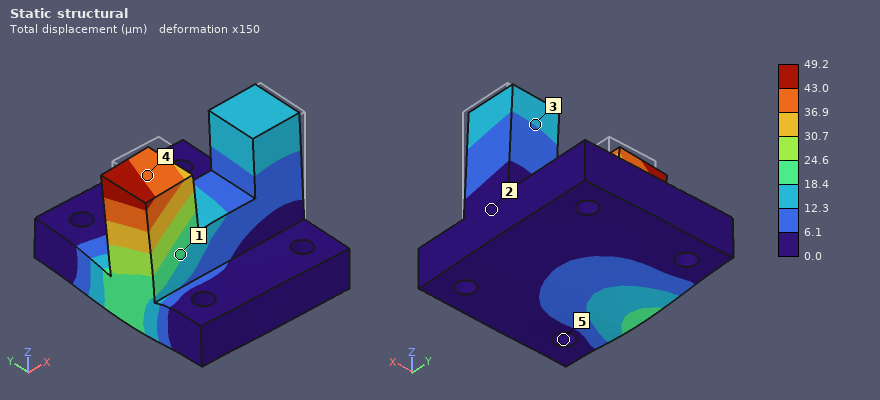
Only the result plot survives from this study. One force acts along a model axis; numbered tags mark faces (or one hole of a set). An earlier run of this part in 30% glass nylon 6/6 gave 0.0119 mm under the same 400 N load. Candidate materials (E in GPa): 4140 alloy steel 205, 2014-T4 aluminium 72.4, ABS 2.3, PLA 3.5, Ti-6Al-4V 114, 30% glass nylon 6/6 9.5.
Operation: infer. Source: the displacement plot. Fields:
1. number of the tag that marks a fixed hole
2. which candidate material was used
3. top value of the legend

5
ABS
49.2 µm
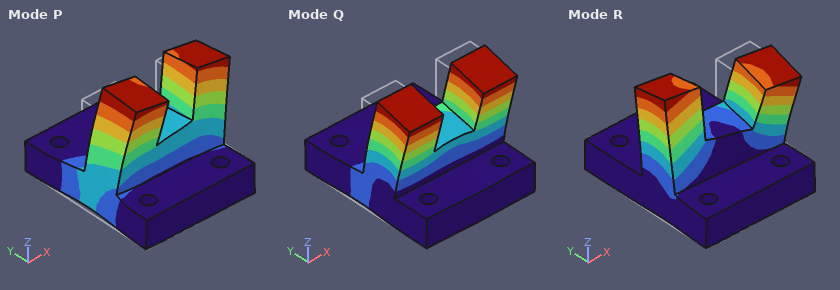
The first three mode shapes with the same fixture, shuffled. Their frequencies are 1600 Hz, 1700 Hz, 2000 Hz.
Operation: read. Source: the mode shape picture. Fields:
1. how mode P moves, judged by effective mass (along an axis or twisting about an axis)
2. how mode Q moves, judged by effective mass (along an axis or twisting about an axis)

along X
along Y
